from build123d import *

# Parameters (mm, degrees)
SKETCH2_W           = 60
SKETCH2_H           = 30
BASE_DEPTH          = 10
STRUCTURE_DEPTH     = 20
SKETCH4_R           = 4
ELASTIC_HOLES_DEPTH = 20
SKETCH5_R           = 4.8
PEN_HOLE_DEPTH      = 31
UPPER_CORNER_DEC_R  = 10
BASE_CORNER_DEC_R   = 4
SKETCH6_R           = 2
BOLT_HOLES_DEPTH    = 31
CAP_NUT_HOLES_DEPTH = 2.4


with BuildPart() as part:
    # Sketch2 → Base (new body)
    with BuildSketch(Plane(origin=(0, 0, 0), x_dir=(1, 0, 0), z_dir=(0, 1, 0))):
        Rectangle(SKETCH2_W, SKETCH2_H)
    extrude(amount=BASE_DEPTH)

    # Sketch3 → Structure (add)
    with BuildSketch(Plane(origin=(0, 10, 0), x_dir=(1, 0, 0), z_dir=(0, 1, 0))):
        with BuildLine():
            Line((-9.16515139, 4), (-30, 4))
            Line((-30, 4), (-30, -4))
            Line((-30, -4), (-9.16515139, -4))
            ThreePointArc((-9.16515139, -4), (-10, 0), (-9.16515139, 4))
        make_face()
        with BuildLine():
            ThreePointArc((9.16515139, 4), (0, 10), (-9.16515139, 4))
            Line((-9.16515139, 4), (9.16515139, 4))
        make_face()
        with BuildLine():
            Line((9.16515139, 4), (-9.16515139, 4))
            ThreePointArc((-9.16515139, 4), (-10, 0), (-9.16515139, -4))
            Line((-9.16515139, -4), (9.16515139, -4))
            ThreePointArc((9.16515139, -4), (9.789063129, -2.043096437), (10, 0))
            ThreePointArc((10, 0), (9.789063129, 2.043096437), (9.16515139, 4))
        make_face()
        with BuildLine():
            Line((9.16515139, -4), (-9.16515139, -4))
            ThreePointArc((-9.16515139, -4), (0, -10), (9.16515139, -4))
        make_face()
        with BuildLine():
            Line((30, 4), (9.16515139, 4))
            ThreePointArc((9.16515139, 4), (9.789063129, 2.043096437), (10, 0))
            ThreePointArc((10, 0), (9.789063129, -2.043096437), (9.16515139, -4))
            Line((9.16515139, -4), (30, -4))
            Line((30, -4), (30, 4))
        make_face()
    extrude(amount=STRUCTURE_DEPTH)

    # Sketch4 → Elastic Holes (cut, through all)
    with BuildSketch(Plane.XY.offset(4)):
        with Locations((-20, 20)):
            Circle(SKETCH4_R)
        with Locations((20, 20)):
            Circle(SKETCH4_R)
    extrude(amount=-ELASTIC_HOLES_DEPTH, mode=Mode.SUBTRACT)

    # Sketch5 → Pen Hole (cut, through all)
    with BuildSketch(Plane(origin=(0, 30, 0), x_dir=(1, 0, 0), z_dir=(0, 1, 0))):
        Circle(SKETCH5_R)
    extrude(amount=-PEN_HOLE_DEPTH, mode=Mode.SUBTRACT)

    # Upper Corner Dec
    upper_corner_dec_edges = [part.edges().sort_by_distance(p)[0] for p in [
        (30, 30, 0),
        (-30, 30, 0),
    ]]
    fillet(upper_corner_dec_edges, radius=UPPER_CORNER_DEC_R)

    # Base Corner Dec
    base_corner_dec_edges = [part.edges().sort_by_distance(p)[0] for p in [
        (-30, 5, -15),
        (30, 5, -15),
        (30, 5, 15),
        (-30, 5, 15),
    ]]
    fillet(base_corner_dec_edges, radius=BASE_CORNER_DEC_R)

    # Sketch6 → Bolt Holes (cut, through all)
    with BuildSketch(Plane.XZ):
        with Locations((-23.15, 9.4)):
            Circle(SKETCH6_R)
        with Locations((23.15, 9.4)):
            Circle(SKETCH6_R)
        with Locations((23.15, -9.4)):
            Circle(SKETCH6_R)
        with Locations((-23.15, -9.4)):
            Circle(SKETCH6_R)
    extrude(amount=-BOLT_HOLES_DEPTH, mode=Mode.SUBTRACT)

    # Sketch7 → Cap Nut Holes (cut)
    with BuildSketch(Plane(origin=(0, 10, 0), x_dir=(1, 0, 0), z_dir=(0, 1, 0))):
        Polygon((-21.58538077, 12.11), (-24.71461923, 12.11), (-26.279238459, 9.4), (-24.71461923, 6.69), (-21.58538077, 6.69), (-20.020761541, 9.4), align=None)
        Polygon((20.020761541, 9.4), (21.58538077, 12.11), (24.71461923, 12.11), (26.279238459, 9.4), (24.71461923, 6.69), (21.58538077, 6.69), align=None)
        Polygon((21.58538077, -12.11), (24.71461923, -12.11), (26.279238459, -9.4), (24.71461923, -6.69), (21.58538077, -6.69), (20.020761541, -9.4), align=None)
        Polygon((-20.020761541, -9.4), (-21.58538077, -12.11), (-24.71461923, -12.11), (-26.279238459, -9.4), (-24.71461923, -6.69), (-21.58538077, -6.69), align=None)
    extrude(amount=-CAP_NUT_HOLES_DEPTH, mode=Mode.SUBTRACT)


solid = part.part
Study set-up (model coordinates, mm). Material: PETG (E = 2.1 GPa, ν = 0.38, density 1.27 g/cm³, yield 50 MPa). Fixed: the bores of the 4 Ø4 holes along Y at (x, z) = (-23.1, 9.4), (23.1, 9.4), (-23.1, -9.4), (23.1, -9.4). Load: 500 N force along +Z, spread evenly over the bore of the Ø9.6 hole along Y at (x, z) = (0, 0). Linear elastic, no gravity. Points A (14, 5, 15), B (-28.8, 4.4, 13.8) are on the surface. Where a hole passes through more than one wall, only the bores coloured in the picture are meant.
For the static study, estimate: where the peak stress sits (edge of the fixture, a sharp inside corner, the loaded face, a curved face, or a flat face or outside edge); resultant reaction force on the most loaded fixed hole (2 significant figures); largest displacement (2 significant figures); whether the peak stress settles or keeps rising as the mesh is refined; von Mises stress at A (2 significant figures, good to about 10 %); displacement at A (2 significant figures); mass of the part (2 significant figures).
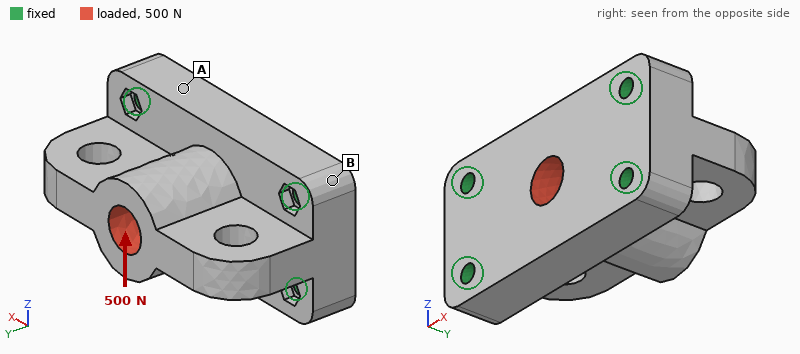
edge of the fixture
220 N
0.14 mm
keeps rising
2.3 MPa
0.027 mm
34 g
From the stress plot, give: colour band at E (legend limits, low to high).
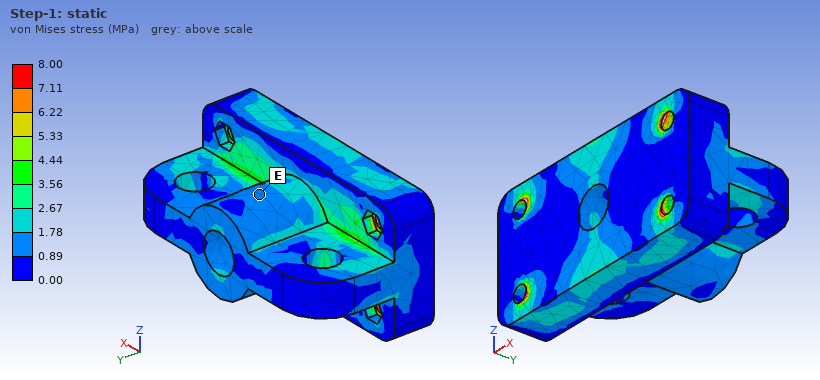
0.89 to 1.78 MPa
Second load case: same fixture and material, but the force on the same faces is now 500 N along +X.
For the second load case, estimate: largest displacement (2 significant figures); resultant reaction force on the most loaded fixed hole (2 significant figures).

29 µm
140 N
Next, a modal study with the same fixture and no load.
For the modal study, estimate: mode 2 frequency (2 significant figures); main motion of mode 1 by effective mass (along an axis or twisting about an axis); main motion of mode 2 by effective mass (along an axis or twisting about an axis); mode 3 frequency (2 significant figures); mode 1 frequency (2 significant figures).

4400 Hz
along Z
along Y
5000 Hz
2800 Hz
